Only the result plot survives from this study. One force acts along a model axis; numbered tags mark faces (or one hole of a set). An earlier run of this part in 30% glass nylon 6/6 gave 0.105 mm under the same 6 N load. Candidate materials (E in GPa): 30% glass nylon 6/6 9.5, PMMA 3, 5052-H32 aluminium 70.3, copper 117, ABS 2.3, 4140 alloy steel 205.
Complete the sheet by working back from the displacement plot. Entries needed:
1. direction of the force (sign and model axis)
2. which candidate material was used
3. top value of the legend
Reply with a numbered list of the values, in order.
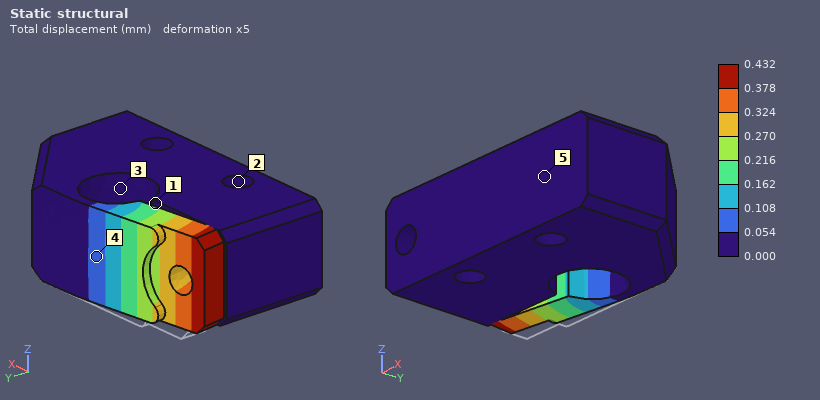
1. -Y
2. ABS
3. 0.432 mm
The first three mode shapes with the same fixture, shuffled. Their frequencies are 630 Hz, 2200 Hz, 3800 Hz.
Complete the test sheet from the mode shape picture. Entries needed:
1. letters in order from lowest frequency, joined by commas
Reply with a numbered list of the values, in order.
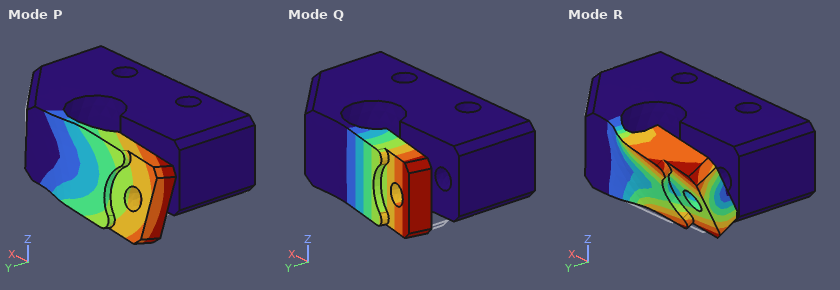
1. Q, P, R
